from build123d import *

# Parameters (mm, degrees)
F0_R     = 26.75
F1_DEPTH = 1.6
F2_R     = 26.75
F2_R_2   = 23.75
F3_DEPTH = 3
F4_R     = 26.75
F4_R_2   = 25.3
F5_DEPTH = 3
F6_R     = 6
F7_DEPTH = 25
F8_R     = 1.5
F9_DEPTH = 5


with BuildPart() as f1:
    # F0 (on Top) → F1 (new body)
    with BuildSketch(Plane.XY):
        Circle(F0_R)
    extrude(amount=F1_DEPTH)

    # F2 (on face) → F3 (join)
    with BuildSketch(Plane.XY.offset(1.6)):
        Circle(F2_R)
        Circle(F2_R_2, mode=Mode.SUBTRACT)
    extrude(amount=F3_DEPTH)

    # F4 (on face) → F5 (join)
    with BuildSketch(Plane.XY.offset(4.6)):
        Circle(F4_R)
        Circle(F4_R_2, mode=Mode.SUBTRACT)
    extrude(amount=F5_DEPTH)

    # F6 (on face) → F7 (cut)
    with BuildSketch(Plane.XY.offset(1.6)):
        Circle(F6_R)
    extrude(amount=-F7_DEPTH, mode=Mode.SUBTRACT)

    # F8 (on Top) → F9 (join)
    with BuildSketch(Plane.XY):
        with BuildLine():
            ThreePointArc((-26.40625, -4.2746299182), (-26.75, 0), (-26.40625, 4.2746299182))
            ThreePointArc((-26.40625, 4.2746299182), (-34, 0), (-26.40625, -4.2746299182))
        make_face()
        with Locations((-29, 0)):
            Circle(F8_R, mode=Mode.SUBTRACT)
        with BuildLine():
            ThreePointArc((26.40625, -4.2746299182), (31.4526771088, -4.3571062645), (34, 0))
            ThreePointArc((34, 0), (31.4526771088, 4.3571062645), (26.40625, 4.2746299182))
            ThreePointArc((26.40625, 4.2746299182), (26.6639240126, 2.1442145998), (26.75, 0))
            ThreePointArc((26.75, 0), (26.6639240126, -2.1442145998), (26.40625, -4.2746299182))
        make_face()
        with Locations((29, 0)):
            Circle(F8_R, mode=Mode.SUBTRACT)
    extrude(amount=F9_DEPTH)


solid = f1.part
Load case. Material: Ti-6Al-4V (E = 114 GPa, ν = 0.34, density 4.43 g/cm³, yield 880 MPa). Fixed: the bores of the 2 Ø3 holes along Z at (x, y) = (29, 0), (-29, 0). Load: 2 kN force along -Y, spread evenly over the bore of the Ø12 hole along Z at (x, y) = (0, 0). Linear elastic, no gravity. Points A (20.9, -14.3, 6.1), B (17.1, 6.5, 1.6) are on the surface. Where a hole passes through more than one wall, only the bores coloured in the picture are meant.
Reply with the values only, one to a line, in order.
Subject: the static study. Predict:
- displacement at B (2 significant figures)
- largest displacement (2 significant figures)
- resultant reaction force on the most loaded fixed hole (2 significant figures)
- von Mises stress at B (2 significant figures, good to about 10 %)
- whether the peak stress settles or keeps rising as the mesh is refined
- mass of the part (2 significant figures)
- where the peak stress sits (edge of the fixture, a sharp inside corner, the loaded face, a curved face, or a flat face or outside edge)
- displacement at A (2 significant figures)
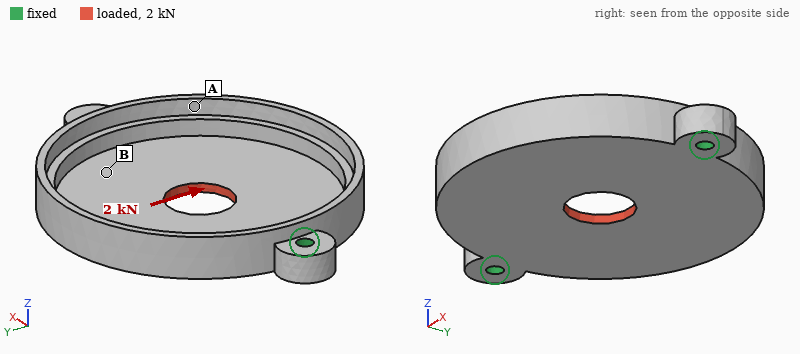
9.7 µm
41 µm
1.0 kN
27 MPa
keeps rising
27 g
edge of the fixture
14 µm
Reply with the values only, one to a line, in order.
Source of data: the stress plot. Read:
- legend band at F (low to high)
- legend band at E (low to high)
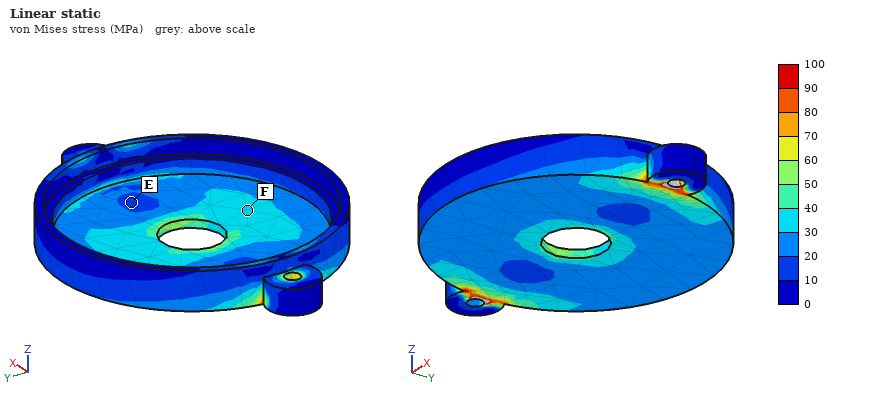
30 to 40 MPa
10 to 20 MPa
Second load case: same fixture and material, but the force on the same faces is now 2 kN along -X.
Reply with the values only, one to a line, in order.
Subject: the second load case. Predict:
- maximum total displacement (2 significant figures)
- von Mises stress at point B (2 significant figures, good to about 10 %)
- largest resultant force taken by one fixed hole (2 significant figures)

9.2 µm
33 MPa
1.0 kN
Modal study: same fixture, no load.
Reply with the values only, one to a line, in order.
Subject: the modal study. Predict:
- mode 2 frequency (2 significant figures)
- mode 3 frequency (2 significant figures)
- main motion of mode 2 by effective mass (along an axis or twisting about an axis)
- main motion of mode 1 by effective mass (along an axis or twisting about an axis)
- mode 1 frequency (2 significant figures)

3900 Hz
7000 Hz
along Z
twisting about X
3300 Hz
